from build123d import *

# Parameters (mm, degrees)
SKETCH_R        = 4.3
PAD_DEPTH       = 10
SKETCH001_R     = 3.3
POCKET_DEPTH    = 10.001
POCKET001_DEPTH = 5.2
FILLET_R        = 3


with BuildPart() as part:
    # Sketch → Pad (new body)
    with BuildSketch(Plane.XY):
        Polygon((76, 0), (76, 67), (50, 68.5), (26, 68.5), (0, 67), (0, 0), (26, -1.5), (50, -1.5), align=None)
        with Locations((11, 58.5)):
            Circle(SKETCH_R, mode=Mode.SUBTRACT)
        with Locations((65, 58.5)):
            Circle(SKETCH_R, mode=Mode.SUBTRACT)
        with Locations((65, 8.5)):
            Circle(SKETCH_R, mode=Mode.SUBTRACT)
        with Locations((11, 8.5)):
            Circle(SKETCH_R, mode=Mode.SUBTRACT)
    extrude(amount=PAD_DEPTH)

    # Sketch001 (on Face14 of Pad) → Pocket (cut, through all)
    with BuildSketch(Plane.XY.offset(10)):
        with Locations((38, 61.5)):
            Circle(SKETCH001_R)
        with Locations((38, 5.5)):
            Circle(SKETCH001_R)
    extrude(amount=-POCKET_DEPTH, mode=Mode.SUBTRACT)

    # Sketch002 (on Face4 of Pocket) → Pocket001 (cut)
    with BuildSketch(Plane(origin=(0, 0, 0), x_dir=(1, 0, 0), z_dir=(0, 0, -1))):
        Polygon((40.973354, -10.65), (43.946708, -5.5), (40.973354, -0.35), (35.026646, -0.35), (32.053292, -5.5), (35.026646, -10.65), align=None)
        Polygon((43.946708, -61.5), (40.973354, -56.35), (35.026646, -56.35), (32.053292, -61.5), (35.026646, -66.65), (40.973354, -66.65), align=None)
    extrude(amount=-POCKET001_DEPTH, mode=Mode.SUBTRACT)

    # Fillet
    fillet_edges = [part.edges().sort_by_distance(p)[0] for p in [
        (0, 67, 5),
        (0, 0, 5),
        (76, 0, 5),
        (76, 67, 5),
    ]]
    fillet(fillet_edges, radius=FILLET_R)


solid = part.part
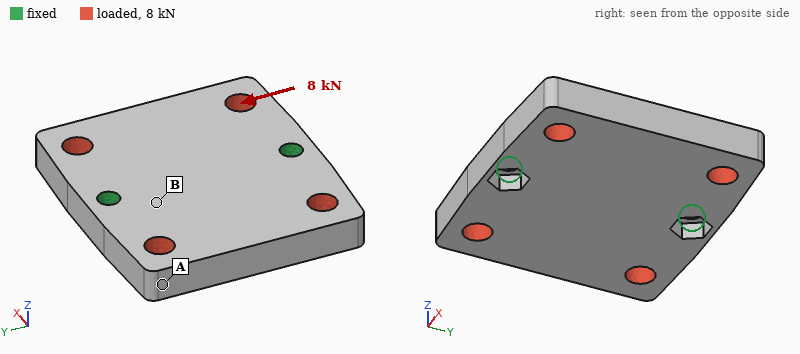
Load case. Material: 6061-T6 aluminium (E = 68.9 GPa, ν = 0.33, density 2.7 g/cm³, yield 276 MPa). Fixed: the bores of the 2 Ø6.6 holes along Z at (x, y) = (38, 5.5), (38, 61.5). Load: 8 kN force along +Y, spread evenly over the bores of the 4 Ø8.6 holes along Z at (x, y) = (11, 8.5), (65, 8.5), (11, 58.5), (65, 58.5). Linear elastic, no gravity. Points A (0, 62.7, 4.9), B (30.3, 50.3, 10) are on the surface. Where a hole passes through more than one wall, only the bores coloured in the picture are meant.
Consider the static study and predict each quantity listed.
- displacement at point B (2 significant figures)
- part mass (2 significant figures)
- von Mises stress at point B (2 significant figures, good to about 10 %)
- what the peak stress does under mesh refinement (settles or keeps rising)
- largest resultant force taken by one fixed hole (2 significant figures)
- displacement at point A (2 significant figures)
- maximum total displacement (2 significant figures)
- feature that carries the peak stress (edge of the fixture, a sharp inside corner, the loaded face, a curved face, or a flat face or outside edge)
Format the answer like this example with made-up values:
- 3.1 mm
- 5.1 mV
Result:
- 5.6 µm
- 130 g
- 21 MPa
- keeps rising
- 4.0 kN
- 15 µm
- 15 µm
- edge of the fixture
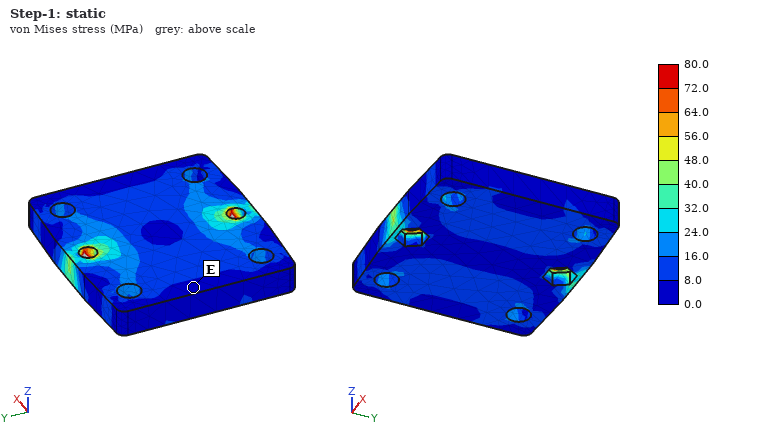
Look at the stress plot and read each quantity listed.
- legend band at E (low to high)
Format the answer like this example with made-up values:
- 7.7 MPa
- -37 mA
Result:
- 0.0 to 8.0 MPa
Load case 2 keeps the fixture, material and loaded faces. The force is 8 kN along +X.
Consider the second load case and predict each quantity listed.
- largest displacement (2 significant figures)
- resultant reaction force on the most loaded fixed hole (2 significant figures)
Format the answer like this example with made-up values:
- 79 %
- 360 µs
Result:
- 50 µm
- 4.0 kN
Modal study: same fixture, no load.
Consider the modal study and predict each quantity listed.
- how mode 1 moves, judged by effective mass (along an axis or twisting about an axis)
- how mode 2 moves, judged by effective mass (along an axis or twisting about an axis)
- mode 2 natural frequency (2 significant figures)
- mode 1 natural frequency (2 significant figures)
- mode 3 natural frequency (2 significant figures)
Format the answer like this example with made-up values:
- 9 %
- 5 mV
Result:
- twisting about Y
- along Z
- 4800 Hz
- 2500 Hz
- 7100 Hz
